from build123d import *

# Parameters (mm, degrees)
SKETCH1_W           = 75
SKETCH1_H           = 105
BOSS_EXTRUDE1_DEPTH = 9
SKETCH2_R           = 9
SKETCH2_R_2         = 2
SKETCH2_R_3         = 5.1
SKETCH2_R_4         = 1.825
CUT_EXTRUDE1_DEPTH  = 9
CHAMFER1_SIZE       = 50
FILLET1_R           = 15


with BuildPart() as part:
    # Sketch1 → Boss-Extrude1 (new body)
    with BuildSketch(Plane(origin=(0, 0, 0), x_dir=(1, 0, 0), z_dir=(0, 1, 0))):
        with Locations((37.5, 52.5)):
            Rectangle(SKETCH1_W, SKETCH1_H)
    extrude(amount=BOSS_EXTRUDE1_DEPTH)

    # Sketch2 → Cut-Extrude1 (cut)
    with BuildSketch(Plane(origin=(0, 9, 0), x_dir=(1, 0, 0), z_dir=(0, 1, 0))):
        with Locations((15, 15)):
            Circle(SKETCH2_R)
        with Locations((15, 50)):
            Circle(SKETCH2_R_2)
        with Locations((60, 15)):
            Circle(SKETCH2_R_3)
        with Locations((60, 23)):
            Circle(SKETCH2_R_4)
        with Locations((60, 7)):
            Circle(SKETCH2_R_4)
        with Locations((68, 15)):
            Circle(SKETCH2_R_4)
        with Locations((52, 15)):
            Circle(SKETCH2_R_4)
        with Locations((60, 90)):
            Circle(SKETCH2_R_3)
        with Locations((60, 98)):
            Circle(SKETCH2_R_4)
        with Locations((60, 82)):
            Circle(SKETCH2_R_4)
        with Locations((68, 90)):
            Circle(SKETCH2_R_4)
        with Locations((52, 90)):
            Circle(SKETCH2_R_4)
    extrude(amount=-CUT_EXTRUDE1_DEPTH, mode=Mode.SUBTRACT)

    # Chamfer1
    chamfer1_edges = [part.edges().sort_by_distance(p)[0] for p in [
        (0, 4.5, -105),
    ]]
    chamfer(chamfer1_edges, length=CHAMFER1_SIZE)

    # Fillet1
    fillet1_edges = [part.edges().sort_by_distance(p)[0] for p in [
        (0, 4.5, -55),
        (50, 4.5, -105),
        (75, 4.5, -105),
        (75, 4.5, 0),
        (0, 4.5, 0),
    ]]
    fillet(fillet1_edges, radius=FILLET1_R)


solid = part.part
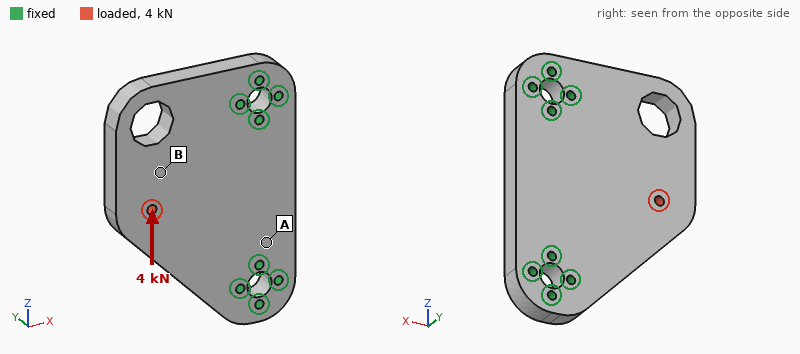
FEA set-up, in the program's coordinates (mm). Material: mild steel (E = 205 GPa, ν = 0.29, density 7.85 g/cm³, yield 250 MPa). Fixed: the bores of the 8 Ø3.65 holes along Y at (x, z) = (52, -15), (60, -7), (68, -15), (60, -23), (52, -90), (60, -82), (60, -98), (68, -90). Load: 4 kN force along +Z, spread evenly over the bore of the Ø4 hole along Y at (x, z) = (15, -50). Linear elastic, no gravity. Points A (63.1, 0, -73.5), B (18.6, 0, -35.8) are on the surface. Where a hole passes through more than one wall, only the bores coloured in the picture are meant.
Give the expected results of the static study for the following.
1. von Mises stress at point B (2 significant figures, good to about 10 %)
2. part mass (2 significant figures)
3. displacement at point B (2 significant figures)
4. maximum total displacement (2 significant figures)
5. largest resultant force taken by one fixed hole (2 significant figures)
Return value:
14 MPa
420 g
3.4 µm
5.1 µm
1.6 kN
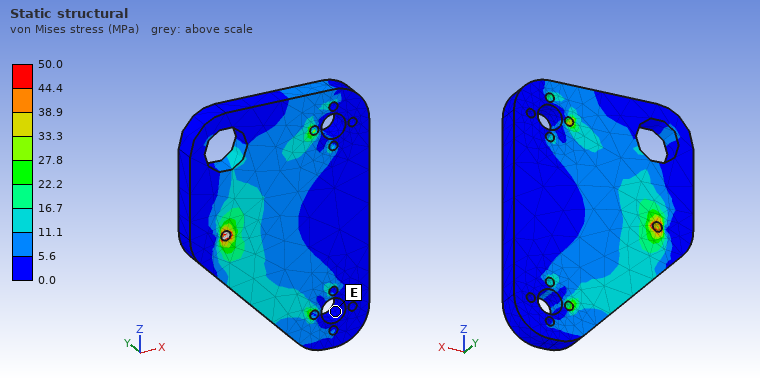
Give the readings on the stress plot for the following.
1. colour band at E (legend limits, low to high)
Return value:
0.0 to 5.6 MPa
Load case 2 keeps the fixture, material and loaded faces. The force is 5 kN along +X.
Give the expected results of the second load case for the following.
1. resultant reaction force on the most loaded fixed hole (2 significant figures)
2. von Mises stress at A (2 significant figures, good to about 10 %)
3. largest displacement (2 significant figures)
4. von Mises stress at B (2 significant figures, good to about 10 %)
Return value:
1.6 kN
7.7 MPa
4.6 µm
9.1 MPa
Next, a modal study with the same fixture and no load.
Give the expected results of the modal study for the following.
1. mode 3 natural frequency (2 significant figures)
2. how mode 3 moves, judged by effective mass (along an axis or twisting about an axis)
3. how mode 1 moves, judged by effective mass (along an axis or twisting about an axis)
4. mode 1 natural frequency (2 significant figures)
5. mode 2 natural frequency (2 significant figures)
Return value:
10 kHz
along Y
along Y
2600 Hz
5800 Hz
